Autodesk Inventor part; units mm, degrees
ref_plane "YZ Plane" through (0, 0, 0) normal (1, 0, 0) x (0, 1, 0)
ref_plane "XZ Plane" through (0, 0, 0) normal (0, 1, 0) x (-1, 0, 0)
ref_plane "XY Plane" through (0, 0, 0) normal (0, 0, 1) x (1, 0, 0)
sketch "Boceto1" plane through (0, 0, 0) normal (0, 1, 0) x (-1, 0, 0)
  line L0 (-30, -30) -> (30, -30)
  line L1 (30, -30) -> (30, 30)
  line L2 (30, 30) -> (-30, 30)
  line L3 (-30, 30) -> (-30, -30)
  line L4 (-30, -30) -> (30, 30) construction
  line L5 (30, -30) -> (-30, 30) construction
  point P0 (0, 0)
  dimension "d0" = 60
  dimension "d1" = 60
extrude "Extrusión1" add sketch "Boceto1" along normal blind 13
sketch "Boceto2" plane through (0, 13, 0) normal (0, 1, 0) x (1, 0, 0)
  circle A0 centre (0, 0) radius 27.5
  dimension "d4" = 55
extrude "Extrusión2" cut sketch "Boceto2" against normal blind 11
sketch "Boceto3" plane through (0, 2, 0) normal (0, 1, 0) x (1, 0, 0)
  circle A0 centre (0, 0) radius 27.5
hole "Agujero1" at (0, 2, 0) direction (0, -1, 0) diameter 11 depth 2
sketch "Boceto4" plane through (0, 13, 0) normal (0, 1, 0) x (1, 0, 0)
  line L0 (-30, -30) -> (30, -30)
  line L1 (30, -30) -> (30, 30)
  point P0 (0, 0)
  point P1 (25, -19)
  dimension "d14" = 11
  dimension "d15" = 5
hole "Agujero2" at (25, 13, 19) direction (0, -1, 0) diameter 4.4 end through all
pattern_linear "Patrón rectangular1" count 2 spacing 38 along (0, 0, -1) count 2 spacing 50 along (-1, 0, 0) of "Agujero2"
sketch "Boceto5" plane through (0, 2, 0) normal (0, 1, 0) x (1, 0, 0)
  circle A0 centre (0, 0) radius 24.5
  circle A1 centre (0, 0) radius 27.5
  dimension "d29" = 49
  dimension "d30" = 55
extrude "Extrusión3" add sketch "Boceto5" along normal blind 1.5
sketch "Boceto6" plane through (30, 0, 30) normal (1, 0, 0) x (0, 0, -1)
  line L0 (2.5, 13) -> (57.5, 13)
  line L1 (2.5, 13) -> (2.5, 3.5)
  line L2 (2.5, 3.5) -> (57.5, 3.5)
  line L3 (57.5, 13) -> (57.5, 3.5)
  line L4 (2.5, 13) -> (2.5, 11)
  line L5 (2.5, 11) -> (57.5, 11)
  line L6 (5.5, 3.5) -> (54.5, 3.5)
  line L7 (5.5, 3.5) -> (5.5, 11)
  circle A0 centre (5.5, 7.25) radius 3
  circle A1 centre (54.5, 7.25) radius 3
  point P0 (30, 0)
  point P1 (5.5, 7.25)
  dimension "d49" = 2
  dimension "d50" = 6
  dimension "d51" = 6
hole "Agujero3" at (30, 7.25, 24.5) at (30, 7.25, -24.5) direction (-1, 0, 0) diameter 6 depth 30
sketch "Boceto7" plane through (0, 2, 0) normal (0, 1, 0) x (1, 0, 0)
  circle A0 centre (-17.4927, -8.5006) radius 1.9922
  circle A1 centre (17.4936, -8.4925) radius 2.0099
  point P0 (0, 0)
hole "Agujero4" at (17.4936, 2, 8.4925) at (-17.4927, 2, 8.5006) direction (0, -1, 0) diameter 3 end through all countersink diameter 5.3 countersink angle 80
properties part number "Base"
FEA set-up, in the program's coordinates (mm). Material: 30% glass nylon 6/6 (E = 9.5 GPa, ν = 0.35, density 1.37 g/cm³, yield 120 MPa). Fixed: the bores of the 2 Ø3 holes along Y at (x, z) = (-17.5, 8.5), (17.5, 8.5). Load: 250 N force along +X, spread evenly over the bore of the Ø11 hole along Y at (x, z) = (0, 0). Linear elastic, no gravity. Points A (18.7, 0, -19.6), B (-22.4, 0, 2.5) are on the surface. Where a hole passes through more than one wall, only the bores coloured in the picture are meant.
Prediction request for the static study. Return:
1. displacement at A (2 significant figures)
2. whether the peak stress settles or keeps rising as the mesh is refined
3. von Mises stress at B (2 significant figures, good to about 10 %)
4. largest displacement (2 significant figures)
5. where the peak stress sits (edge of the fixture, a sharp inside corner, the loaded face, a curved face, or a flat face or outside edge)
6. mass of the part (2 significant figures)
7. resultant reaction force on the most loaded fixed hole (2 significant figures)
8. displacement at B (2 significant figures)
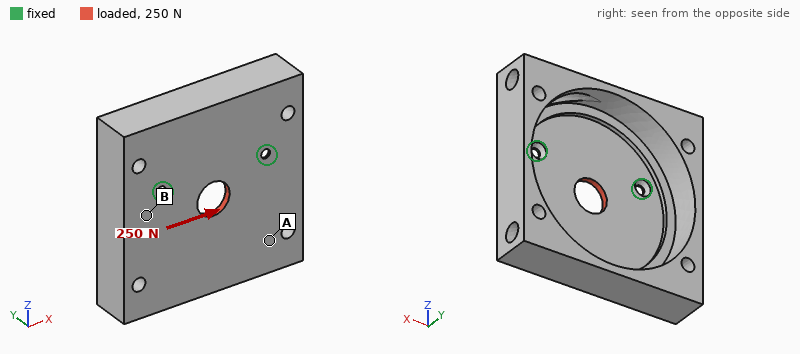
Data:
17 µm
keeps rising
2.6 MPa
23 µm
edge of the fixture
27 g
140 N
9.1 µm
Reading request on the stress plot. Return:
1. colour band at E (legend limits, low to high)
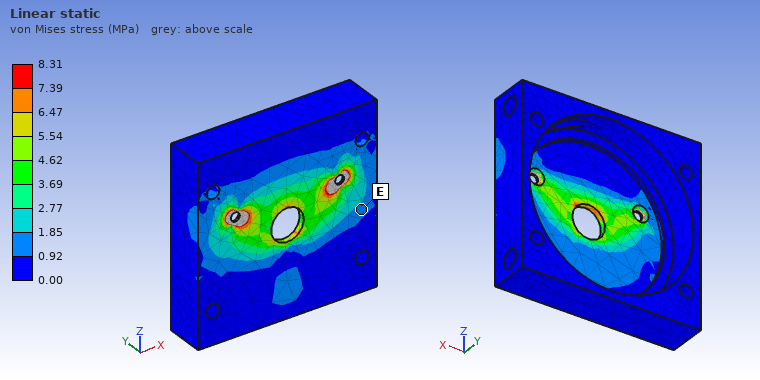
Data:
0.92 to 1.85 MPa
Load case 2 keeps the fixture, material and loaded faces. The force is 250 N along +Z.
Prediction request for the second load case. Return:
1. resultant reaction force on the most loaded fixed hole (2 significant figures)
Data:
130 N
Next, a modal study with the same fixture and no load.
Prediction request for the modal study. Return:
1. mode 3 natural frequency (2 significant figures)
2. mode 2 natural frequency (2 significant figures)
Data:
1700 Hz
1300 Hz
